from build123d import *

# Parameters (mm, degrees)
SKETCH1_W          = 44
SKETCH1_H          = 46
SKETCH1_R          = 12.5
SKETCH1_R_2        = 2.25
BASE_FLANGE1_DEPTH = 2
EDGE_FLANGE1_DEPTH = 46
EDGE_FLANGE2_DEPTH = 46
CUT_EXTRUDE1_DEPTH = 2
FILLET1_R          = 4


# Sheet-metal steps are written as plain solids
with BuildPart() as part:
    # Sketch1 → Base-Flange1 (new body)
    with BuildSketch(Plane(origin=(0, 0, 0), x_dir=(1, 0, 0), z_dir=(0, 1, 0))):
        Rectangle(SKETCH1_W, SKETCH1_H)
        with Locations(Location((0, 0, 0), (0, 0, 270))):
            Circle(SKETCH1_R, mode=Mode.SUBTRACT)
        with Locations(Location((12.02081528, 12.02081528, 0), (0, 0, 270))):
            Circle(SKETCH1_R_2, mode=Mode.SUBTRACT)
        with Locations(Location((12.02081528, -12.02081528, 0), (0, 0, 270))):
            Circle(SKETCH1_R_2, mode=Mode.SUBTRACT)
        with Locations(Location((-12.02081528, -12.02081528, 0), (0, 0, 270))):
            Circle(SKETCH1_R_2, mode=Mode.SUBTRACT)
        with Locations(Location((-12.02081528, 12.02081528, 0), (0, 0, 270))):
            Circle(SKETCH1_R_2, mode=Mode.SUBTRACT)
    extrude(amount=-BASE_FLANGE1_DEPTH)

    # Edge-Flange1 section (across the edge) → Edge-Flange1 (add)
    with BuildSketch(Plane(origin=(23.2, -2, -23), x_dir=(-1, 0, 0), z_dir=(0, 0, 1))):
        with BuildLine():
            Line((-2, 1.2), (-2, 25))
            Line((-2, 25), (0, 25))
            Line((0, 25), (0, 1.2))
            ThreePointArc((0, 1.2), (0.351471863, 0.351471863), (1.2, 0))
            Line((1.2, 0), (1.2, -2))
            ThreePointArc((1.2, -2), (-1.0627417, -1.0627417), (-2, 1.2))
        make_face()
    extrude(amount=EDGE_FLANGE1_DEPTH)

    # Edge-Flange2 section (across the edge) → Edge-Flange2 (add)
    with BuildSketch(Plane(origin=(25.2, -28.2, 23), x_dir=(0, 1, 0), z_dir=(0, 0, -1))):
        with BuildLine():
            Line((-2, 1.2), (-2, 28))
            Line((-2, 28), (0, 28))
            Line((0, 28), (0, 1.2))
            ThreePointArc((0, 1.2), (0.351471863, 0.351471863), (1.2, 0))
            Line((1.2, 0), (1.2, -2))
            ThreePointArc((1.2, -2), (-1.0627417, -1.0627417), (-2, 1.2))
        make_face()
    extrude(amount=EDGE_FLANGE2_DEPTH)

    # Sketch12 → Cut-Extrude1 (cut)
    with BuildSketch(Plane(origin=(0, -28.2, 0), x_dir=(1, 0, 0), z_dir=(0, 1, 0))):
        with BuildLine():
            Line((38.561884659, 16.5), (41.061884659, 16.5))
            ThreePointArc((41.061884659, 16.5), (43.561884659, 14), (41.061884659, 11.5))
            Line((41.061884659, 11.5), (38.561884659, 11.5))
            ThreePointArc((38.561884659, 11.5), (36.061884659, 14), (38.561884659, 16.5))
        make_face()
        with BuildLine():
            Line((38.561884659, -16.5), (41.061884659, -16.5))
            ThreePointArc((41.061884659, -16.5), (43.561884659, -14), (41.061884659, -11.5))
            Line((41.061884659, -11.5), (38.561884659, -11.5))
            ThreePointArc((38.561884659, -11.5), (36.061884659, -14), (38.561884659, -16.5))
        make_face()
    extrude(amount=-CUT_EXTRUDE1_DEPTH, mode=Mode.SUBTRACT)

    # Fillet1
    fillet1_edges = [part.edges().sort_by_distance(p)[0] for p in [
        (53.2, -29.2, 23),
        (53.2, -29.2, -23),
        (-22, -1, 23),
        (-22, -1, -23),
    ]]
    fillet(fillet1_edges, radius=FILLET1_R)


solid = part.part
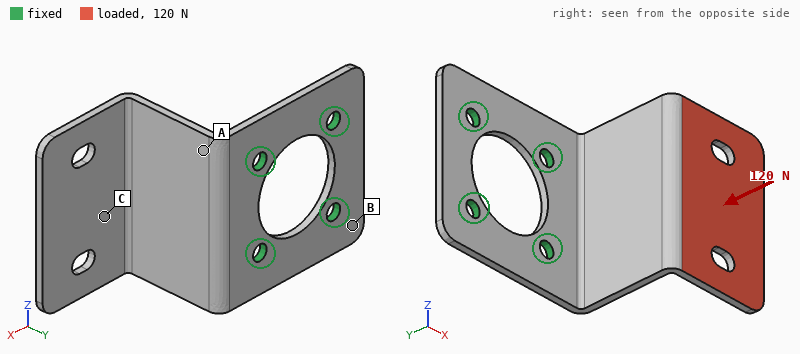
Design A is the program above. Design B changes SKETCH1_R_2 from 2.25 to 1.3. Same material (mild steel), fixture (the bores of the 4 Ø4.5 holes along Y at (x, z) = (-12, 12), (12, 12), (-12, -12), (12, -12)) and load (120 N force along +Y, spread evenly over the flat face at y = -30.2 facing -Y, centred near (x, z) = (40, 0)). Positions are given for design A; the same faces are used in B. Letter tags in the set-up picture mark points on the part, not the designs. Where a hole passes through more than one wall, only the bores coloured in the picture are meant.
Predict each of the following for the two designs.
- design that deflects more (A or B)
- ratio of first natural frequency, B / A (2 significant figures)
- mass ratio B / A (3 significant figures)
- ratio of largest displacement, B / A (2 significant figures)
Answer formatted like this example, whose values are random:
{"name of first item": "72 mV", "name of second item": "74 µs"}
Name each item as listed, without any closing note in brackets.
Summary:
{"design that deflects more": "B", "ratio of first natural frequency, B / A": "0.95", "mass ratio B / A": "1.01", "ratio of largest displacement, B / A": "1.1"}
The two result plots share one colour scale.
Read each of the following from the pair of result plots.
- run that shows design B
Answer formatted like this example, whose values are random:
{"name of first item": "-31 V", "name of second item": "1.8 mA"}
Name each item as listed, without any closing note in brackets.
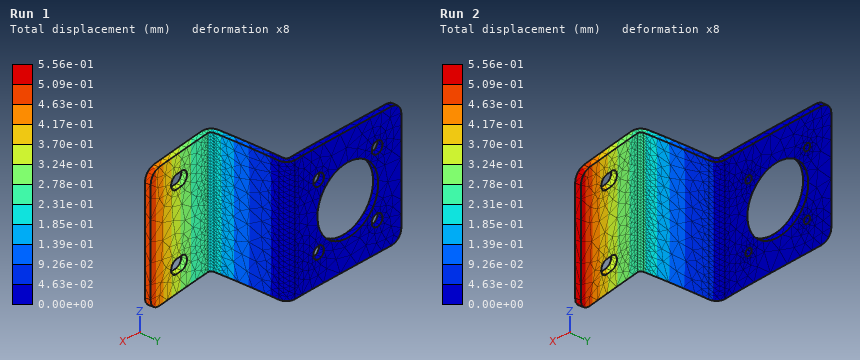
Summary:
{"run that shows design B": "Run 2"}
